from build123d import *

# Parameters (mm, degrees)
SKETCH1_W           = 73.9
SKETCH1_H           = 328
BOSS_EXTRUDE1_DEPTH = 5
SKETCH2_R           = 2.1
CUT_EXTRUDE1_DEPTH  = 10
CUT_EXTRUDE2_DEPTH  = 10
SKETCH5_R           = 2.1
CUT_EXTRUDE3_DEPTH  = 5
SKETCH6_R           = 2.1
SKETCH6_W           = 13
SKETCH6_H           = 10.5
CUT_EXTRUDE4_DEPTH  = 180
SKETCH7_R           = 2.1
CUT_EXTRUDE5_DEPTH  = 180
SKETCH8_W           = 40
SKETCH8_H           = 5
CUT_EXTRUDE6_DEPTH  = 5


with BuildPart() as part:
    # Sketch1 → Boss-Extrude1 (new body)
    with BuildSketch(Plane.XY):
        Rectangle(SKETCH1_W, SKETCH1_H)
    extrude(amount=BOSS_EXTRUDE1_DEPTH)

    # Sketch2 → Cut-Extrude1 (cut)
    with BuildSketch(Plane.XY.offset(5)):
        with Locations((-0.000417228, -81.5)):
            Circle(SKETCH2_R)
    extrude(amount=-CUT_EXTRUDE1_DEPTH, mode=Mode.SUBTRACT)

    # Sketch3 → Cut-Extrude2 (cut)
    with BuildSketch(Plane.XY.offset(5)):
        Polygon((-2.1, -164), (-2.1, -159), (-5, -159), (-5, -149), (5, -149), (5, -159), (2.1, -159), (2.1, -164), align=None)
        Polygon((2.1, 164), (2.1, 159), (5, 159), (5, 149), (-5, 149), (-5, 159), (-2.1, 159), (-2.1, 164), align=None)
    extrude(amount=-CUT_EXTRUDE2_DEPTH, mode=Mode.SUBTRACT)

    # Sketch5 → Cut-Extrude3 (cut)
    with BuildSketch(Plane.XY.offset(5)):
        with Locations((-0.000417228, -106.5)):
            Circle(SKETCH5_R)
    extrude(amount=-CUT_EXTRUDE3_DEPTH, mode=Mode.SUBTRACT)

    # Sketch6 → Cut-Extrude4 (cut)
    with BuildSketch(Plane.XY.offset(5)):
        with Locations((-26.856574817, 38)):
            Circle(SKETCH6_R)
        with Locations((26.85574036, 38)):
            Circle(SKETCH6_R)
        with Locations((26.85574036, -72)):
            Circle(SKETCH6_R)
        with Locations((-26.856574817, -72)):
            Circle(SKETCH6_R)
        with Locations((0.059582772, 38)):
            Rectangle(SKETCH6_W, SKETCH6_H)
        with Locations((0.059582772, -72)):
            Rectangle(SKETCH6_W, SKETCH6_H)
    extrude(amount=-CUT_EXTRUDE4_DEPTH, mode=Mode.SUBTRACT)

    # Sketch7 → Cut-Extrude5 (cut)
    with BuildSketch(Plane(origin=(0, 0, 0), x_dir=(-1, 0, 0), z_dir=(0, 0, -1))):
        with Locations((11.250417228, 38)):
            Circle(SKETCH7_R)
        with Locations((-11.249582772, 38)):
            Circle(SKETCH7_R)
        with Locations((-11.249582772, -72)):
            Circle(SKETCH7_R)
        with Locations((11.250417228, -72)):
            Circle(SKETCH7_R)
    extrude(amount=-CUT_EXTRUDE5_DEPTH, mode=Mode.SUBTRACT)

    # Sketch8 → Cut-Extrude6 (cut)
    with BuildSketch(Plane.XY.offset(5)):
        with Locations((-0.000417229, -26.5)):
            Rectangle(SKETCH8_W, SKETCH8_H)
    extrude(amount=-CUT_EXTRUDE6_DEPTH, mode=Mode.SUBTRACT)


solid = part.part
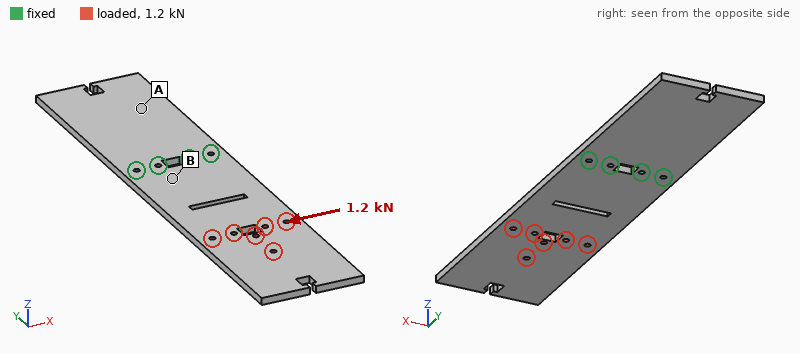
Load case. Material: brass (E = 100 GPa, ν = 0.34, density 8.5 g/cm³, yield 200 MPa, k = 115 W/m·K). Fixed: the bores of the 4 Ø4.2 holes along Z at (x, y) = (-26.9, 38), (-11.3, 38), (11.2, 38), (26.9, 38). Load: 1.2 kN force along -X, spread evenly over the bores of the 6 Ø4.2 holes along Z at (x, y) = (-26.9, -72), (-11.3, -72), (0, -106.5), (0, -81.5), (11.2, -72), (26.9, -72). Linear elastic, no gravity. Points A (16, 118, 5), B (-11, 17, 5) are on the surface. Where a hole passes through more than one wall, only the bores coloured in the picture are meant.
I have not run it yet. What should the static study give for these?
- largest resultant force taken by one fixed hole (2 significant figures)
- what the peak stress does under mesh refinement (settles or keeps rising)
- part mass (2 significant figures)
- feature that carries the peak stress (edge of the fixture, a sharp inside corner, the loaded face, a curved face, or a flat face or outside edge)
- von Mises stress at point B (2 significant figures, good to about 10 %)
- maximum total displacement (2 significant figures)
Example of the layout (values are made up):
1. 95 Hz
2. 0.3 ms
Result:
1. 2.3 kN
2. keeps rising
3. 990 g
4. edge of the fixture
5. 12 MPa
6. 0.11 mm
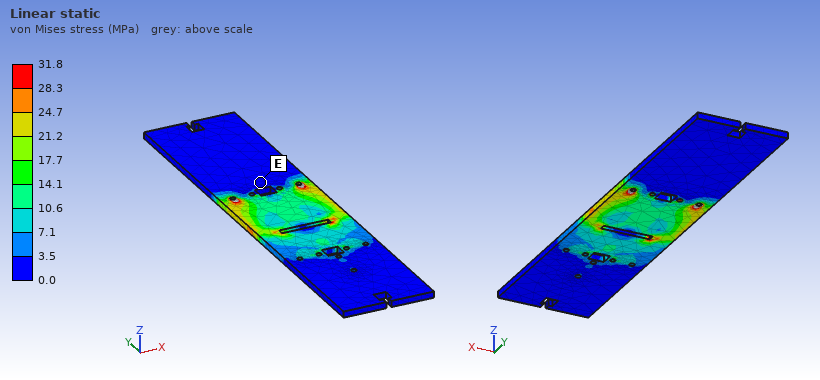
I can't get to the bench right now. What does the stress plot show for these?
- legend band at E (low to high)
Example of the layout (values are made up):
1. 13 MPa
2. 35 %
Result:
1. 0.0 to 3.5 MPa
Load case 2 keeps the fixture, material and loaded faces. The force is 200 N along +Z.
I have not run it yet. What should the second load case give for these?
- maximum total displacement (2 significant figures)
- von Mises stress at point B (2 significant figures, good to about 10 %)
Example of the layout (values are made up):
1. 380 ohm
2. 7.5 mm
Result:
1. 3.4 mm
2. 55 MPa
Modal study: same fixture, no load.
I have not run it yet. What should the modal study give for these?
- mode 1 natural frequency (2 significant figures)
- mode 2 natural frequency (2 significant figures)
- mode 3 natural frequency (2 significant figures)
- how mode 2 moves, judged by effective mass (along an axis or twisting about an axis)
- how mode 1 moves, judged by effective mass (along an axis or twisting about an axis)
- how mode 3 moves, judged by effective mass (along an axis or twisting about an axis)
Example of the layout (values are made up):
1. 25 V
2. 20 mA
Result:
1. 64 Hz
2. 180 Hz
3. 370 Hz
4. along Z
5. along Z
6. twisting about Y
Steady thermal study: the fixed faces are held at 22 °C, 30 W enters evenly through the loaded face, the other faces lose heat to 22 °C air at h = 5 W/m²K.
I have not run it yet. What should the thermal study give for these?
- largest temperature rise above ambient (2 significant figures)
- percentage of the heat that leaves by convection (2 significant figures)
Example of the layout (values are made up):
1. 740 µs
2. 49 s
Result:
1. 81 K
2. 29 %
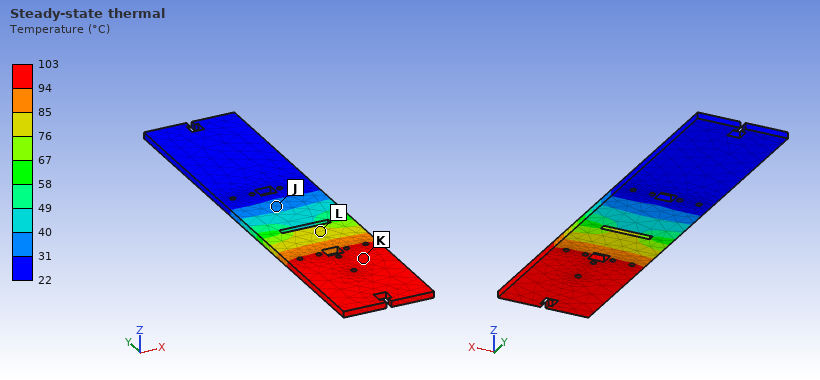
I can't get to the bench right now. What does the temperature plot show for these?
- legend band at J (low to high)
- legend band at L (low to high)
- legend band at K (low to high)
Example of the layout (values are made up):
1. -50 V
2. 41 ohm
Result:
1. 31 to 40 °C
2. 76 to 85 °C
3. 94 to 103 °C
